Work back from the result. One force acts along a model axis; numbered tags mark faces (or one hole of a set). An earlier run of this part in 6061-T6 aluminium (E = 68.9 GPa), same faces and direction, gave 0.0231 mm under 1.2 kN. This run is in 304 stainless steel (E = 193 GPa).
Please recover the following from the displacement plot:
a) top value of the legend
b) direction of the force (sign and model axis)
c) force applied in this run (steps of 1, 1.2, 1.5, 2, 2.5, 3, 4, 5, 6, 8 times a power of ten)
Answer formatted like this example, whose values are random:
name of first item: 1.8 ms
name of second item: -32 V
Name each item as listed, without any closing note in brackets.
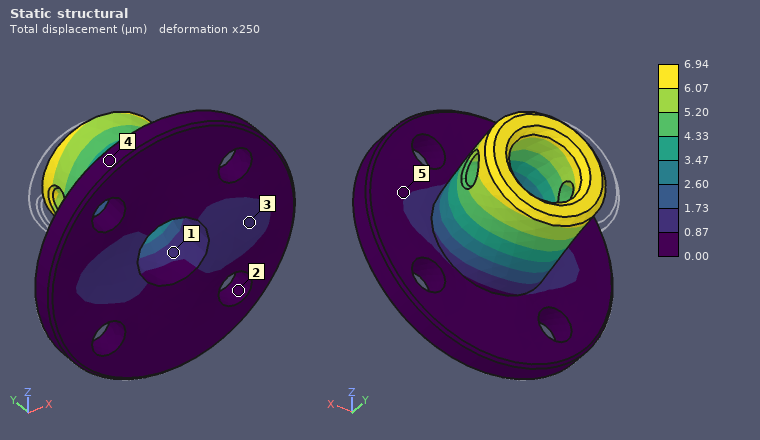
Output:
top value of the legend: 6.94 µm
direction of the force: +X
force applied in this run: 1 kN
